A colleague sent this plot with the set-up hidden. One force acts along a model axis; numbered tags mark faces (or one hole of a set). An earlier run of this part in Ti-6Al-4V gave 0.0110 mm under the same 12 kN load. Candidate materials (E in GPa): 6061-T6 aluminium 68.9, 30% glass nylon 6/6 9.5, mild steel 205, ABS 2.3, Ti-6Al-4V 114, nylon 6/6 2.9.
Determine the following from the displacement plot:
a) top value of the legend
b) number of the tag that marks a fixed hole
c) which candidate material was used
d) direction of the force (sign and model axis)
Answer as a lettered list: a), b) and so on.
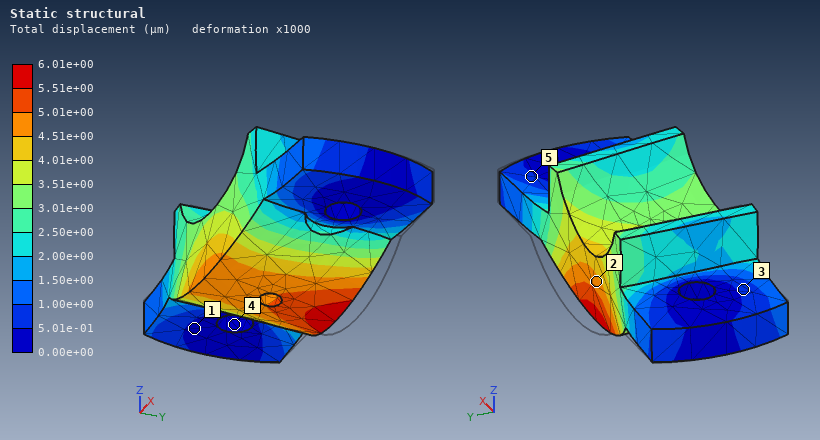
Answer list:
a) 6.01e+00 µm
b) 4
c) mild steel
d) -Y
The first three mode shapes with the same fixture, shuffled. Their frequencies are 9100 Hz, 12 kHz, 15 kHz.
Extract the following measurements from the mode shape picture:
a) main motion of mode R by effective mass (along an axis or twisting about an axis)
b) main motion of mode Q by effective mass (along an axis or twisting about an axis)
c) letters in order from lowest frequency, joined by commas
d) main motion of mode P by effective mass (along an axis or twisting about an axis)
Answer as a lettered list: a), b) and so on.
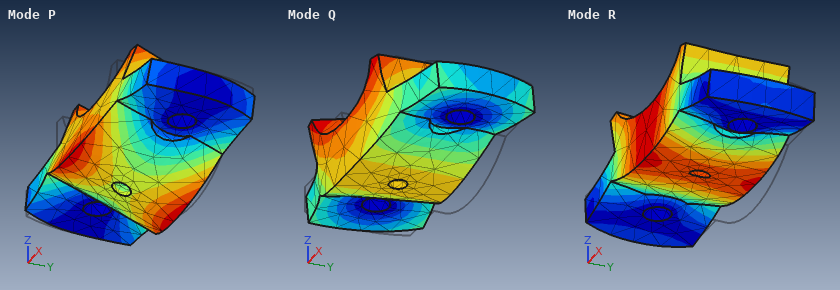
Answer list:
a) along Z
b) along Y
c) P, R, Q
d) twisting about X
